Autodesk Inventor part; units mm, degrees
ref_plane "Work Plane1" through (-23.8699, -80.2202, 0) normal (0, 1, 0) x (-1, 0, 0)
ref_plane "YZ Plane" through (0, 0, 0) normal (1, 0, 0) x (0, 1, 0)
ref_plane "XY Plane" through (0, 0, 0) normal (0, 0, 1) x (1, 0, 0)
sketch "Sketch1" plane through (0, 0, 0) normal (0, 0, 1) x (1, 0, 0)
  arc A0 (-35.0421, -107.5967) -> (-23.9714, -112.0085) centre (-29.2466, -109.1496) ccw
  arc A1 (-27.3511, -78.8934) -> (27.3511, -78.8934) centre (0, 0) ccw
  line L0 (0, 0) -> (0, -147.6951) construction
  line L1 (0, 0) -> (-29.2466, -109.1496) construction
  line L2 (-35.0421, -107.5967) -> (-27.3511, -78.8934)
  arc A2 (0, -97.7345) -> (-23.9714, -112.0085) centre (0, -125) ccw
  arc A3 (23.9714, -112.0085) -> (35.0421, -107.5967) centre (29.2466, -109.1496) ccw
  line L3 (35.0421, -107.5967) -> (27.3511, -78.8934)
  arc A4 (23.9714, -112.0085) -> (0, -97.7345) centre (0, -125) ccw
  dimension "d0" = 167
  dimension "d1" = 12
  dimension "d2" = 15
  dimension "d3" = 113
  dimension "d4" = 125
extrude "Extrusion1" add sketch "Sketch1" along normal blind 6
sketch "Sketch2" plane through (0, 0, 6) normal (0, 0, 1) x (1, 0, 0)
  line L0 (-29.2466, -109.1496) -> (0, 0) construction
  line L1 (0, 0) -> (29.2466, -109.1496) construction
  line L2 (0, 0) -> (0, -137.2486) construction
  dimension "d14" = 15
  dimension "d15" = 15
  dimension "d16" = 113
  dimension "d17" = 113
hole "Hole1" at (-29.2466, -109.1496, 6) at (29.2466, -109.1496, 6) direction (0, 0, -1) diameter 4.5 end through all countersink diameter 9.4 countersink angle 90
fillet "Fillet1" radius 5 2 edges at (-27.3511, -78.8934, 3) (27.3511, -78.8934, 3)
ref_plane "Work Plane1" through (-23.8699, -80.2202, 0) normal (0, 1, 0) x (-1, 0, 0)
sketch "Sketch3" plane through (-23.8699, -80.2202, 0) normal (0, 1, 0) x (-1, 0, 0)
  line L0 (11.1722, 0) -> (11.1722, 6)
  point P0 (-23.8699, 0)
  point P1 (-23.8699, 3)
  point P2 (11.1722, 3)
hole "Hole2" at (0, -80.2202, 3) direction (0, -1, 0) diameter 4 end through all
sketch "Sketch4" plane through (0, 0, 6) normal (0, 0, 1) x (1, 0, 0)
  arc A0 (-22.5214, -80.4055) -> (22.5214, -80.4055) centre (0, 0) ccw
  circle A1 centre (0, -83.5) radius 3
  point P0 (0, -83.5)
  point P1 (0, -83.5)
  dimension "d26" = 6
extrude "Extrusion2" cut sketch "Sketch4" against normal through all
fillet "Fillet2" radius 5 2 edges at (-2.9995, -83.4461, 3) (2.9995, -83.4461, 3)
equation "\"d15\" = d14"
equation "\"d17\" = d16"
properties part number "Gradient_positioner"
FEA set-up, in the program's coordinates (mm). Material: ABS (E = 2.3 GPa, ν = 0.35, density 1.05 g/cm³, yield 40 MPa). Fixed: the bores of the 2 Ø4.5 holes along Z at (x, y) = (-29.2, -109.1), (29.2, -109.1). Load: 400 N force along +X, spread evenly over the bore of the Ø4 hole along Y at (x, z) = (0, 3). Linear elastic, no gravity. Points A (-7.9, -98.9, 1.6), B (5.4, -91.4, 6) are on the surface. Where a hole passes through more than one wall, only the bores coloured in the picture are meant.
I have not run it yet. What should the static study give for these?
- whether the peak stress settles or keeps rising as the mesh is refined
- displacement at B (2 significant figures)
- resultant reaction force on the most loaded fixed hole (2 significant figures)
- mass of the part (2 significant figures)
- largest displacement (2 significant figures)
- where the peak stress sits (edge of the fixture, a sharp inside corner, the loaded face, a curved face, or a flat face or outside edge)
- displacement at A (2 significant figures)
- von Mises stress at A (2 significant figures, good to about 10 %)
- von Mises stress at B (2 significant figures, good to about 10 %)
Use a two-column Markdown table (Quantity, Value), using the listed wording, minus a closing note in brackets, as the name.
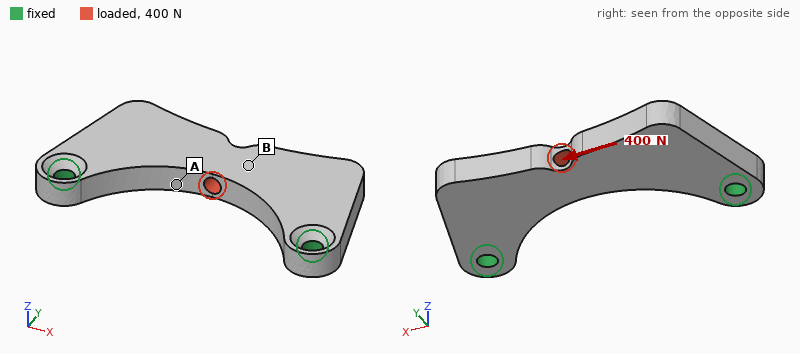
| Quantity | Value |
|---|---|
| whether the peak stress settles or keeps rising as the mesh is refined | keeps rising |
| displacement at B | 81 µm |
| resultant reaction force on the most loaded fixed hole | 220 N |
| mass of the part | 8.7 g |
| largest displacement | 97 µm |
| where the peak stress sits | edge of the fixture |
| displacement at A | 79 µm |
| von Mises stress at A | 7.5 MPa |
| von Mises stress at B | 3.4 MPa |
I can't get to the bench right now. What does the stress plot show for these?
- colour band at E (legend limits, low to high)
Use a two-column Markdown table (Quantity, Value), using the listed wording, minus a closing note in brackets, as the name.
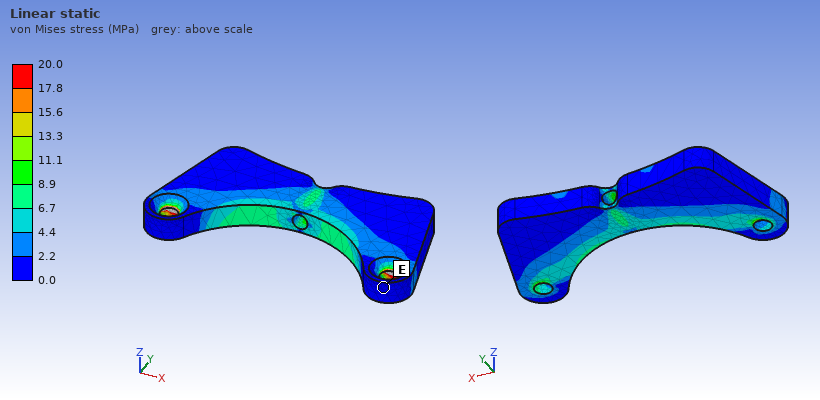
| Quantity | Value |
|---|---|
| colour band at E | 0.0 to 2.2 MPa |
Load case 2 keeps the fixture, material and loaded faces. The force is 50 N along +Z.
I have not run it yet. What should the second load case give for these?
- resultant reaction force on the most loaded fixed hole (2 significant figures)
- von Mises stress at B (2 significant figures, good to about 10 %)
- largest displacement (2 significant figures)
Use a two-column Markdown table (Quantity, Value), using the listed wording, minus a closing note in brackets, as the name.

| Quantity | Value |
|---|---|
| resultant reaction force on the most loaded fixed hole | 25 N |
| von Mises stress at B | 3.6 MPa |
| largest displacement | 0.37 mm |
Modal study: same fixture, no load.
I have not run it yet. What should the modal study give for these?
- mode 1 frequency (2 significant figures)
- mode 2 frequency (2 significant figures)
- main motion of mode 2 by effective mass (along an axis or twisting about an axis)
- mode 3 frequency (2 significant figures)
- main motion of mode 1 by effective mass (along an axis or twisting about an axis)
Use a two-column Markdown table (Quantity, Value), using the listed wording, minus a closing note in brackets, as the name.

| Quantity | Value |
|---|---|
| mode 1 frequency | 980 Hz |
| mode 2 frequency | 2000 Hz |
| main motion of mode 2 by effective mass | twisting about Y |
| mode 3 frequency | 3100 Hz |
| main motion of mode 1 by effective mass | along Z |
